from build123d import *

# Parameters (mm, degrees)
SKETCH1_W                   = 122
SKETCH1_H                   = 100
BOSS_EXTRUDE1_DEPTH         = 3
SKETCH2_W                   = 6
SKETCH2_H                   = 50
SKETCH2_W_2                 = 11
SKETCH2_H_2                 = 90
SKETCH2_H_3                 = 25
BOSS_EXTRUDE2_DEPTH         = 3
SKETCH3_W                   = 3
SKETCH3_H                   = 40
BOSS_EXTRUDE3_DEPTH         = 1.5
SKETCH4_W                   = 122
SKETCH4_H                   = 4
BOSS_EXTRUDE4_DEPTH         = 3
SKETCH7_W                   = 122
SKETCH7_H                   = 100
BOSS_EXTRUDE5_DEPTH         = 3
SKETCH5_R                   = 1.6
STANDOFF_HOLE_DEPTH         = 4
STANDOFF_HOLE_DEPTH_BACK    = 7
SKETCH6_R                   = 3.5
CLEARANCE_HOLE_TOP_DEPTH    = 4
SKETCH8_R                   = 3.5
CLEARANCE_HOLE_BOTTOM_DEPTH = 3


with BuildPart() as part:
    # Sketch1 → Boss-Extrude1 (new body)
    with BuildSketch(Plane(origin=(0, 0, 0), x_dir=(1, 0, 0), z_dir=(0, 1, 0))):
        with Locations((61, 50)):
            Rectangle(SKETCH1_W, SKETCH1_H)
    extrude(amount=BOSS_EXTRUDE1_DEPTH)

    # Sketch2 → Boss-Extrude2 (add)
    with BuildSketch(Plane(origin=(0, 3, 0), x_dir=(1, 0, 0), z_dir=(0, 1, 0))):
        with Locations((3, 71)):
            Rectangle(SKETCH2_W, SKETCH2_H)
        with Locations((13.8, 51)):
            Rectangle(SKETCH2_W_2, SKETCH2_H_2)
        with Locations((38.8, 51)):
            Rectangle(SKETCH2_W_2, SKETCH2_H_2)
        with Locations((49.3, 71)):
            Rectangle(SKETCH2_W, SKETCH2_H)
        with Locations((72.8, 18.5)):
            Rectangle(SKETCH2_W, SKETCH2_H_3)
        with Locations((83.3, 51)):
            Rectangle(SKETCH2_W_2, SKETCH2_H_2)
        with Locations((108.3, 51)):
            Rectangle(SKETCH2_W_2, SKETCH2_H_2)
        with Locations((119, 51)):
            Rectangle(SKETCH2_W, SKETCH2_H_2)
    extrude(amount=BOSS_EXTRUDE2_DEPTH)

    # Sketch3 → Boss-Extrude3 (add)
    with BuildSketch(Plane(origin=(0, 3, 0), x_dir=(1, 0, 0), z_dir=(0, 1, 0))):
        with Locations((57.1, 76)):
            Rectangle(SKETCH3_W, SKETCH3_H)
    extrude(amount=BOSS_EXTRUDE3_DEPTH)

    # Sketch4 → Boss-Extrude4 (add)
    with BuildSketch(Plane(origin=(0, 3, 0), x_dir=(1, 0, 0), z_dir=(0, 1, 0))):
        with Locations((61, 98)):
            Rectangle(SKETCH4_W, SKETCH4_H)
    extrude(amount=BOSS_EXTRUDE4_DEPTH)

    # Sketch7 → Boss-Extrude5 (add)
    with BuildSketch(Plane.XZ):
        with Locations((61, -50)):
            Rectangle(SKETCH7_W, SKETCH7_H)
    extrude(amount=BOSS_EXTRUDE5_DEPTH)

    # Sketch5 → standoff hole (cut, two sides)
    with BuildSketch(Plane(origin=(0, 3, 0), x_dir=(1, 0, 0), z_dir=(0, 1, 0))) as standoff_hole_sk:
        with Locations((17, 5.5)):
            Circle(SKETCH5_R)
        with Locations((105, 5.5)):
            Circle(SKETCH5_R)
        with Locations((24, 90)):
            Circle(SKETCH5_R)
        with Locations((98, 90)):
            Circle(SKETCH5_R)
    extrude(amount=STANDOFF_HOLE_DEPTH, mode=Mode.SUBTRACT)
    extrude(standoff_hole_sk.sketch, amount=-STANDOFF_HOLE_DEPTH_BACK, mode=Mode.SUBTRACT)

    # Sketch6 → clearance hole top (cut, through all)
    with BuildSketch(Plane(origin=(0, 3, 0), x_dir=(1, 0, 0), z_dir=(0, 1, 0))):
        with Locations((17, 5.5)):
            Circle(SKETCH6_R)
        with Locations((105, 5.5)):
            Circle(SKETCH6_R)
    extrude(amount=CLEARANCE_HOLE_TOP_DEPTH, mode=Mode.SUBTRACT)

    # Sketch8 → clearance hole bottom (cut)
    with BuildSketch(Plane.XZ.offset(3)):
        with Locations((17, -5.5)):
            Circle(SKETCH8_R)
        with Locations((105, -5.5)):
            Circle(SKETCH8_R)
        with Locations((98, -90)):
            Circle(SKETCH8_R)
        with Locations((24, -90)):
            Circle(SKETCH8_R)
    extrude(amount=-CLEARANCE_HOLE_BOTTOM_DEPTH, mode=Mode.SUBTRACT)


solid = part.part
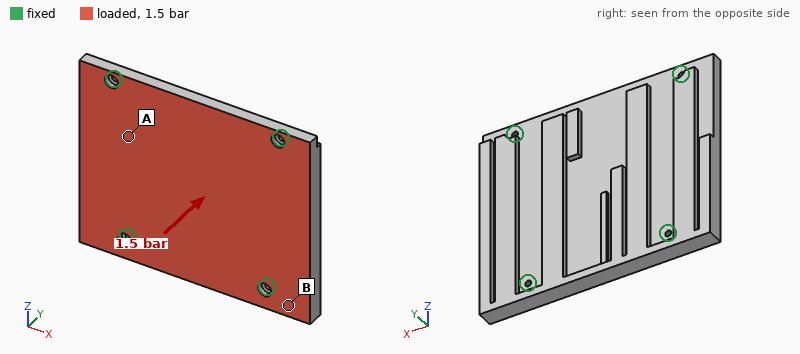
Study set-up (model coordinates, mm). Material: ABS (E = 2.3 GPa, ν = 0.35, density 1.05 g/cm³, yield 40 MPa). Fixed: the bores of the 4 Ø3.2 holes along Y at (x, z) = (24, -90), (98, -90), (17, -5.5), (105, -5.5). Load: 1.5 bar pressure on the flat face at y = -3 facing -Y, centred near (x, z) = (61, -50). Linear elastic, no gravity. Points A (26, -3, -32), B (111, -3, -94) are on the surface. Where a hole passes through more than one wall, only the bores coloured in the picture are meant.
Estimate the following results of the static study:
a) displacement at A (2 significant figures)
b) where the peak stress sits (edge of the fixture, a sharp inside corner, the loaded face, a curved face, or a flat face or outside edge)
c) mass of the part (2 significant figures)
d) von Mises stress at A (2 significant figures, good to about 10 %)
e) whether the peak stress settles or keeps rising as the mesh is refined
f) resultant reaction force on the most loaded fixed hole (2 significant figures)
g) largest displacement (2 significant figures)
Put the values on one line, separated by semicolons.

0.89 mm; edge of the fixture; 94 g; 9.9 MPa; keeps rising; 540 N; 1.4 mm
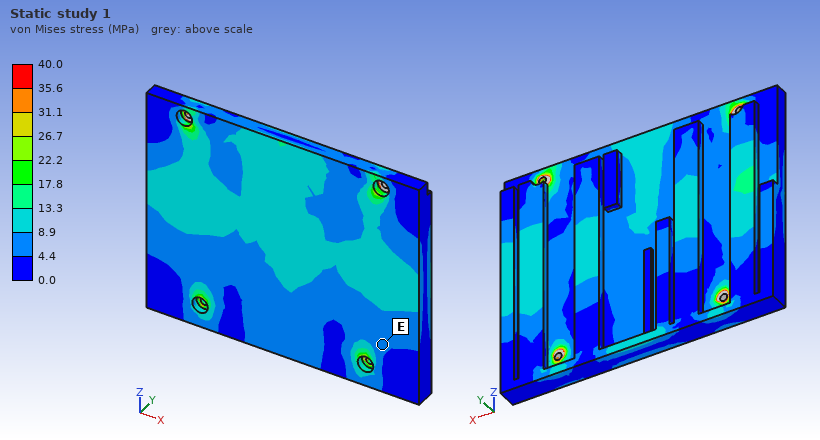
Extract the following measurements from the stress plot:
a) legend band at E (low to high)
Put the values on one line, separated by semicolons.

4.4 to 8.9 MPa
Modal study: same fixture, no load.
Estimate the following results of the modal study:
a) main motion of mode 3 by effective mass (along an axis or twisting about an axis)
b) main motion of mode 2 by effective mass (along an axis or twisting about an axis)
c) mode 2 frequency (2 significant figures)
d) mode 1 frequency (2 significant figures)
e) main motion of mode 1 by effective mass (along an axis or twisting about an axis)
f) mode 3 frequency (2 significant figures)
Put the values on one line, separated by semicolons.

twisting about Z; along Y; 890 Hz; 700 Hz; along Y; 950 Hz
